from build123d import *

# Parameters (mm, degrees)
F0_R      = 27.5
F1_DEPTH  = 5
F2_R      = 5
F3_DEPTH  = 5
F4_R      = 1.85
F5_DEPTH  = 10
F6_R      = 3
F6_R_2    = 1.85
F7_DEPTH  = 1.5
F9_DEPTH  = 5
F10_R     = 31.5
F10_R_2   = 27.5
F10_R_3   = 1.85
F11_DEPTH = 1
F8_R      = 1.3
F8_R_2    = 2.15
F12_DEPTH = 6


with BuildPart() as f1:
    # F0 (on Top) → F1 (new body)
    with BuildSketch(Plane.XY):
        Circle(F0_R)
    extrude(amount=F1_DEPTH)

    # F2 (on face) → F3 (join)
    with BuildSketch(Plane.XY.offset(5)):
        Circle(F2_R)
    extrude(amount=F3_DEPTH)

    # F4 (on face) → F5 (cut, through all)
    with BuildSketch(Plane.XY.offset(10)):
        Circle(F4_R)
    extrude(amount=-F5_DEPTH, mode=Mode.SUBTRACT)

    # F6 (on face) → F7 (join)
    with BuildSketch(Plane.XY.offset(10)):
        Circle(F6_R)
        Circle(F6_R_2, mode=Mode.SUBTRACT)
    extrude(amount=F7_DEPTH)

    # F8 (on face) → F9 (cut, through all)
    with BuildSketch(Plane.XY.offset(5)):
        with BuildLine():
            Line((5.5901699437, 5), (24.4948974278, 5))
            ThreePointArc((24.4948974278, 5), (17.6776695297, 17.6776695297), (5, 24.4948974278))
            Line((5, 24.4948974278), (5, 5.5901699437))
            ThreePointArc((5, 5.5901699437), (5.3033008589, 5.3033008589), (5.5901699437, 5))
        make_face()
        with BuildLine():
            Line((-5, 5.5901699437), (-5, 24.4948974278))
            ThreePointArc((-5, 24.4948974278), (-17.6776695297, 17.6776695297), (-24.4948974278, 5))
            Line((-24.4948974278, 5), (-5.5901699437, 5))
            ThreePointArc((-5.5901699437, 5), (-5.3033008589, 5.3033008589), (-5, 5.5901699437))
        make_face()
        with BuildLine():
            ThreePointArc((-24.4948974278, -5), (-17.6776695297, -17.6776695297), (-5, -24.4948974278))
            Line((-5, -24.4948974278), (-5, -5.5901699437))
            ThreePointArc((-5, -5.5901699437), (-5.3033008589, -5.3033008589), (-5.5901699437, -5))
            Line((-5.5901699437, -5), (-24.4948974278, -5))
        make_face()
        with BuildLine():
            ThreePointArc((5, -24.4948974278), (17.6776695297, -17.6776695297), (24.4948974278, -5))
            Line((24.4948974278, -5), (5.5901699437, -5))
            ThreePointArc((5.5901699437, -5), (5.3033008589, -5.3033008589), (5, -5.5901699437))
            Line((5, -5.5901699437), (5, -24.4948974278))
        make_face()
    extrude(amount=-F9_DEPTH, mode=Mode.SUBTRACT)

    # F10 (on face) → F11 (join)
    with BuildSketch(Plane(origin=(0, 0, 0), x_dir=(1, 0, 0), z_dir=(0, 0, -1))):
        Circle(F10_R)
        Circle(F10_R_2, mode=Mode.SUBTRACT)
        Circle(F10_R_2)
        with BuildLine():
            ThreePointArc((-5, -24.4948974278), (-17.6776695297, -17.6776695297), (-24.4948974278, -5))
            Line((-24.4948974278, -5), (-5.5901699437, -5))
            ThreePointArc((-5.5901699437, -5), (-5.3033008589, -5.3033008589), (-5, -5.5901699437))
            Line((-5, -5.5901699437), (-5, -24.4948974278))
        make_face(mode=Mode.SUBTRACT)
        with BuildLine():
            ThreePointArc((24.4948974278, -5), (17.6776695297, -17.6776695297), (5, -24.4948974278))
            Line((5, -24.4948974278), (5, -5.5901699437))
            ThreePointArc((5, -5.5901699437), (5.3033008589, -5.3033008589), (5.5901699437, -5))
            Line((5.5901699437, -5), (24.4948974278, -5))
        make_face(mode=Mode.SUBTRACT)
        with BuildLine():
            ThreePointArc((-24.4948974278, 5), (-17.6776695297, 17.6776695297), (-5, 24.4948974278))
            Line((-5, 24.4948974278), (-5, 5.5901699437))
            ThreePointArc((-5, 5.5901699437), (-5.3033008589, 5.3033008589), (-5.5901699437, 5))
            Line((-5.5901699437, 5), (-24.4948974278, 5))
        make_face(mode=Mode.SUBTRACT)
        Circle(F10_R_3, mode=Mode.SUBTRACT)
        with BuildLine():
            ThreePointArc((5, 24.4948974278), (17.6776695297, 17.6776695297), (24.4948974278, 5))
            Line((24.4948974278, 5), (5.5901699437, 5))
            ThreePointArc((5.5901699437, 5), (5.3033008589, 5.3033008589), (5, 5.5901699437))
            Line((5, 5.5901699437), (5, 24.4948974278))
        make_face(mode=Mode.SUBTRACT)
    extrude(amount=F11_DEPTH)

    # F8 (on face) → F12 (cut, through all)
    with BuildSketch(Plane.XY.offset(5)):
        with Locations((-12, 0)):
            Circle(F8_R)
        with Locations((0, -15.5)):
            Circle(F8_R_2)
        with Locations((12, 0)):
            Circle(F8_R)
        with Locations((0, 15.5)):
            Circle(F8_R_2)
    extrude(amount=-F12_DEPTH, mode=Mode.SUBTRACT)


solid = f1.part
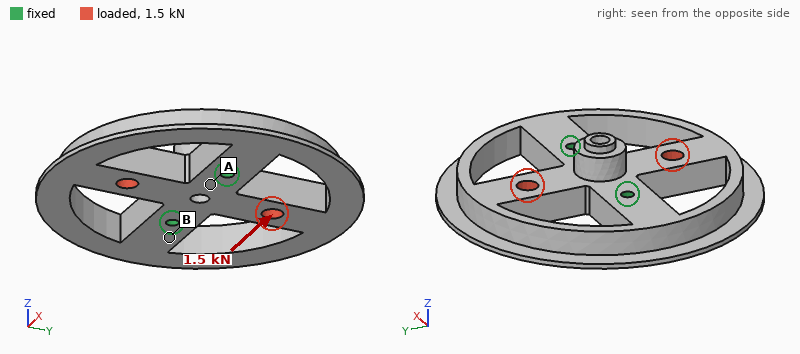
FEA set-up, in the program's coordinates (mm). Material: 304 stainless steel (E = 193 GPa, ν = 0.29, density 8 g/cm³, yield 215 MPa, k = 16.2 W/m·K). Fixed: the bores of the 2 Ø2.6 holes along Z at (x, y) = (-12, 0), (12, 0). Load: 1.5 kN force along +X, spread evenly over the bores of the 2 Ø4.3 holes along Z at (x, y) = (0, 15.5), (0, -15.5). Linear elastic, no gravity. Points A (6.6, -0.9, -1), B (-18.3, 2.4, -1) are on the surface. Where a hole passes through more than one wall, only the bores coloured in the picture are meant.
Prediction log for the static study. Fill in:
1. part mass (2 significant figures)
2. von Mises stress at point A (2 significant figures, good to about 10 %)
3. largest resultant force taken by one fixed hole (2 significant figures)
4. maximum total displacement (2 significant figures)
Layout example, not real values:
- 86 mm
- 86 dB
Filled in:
- 69 g
- 10 MPa
- 750 N
- 5.9 µm
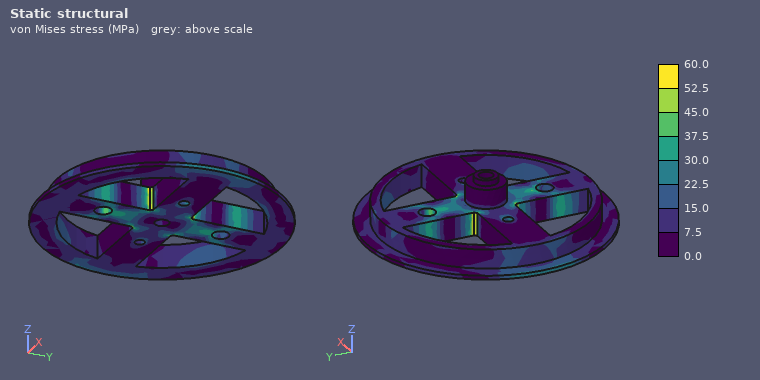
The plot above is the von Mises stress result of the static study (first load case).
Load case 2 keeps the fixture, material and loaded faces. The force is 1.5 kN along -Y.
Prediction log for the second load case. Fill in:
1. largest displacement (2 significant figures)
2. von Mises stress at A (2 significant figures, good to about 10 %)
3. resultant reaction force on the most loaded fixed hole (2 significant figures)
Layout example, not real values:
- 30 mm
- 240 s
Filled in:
- 2.8 µm
- 24 MPa
- 750 N
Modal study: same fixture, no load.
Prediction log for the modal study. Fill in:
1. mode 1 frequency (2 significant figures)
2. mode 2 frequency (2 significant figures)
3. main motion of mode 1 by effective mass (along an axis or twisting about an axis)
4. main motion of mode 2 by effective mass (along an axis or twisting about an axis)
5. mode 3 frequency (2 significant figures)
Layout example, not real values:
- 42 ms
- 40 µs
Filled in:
- 3800 Hz
- 5300 Hz
- twisting about X
- along Z
- 7900 Hz
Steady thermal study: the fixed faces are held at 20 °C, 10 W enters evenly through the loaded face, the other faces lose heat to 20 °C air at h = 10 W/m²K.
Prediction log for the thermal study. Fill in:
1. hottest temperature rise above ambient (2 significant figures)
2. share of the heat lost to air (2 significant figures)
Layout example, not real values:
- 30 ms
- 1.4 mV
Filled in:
- 73 K
- 23 %
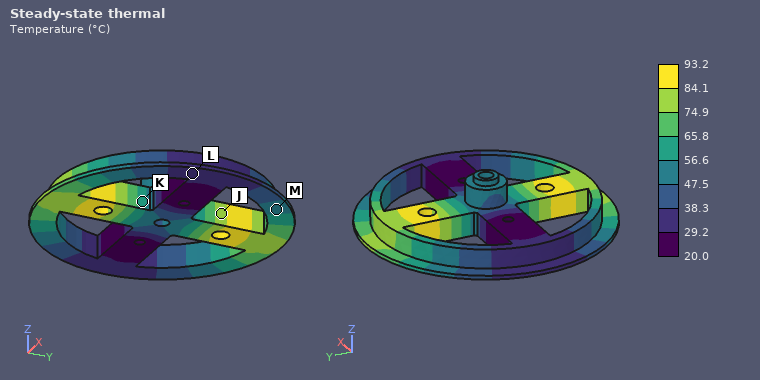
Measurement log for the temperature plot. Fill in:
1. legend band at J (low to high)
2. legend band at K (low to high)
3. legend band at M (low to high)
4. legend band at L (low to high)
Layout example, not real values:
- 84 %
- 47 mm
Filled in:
- 74.9 to 84.1 °C
- 56.6 to 65.8 °C
- 47.5 to 56.6 °C
- 29.2 to 38.3 °C
